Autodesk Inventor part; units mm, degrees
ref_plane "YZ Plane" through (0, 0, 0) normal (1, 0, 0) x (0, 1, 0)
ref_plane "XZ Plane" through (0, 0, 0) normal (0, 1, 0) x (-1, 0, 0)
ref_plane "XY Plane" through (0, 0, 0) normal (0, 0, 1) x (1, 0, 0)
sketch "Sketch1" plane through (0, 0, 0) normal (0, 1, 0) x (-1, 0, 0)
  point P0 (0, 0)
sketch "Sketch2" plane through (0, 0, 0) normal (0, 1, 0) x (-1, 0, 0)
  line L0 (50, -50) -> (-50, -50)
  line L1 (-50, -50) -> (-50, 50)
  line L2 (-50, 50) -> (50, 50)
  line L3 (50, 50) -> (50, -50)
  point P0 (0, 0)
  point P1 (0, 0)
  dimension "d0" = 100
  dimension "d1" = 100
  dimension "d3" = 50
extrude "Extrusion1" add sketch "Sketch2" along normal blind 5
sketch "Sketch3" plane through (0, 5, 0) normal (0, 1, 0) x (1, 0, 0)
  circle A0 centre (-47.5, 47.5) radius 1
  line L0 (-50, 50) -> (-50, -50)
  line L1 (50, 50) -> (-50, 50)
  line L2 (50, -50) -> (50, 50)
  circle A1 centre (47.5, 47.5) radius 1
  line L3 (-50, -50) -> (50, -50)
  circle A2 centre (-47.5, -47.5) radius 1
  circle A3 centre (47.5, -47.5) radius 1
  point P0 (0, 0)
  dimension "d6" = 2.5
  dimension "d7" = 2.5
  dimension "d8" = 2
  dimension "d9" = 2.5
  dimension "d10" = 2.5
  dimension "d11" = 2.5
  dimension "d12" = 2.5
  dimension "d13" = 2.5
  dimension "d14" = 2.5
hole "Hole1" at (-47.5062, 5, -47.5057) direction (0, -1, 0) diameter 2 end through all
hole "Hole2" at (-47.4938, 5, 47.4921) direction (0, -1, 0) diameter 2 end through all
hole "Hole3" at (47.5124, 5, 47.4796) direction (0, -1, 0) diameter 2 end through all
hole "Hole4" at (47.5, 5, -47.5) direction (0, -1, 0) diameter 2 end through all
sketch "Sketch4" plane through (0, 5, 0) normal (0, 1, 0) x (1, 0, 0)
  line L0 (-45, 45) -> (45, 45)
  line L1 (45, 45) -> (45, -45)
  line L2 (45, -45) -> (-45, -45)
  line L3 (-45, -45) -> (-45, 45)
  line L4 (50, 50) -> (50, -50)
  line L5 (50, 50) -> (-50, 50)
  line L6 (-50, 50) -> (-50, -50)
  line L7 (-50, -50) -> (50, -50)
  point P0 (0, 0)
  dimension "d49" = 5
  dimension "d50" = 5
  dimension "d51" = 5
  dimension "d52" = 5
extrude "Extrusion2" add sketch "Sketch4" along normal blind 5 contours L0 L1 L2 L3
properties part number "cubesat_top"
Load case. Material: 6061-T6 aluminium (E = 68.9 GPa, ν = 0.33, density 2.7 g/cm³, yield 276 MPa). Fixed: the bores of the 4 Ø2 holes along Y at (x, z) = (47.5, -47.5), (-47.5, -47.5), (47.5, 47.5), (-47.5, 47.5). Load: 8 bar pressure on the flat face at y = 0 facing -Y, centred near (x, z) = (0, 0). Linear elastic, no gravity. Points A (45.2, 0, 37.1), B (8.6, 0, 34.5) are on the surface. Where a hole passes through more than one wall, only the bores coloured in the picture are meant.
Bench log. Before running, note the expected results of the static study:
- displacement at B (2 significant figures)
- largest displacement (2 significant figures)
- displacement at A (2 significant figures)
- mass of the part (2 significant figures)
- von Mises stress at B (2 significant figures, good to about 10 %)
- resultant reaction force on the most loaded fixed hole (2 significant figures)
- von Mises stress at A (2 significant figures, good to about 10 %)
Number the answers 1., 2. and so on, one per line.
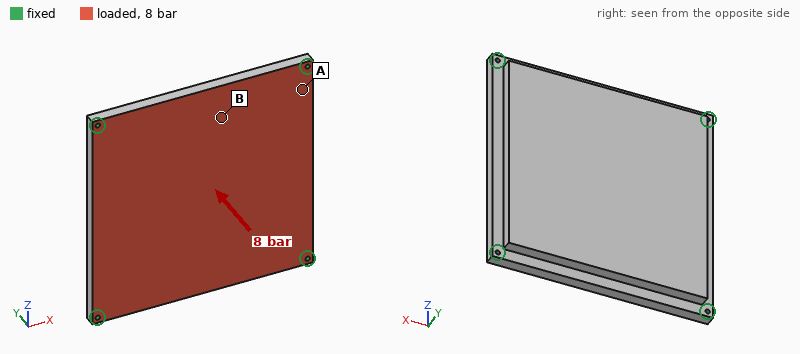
1. 0.16 mm
2. 0.20 mm
3. 0.060 mm
4. 240 g
5. 35 MPa
6. 3.2 kN
7. 20 MPa
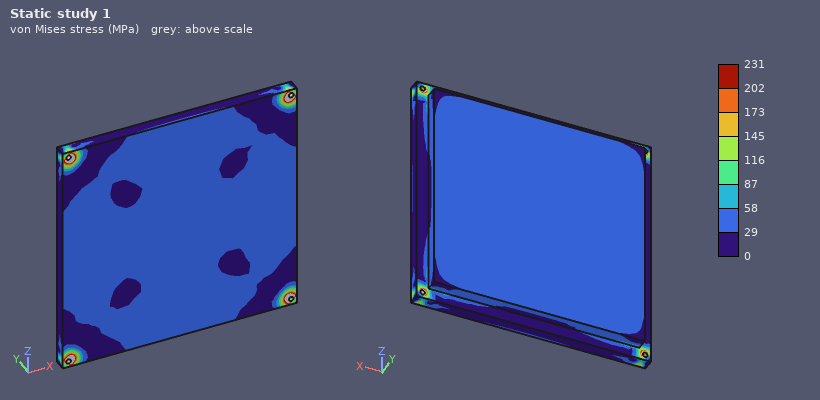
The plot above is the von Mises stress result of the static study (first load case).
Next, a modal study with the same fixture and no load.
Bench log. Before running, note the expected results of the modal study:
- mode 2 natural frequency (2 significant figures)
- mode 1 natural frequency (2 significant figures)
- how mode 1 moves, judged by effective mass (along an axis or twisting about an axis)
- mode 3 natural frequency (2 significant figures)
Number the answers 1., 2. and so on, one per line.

1. 4100 Hz
2. 2200 Hz
3. along Y
4. 4100 Hz
